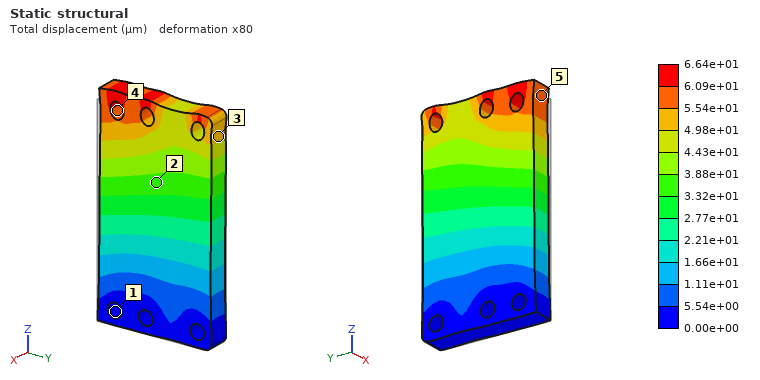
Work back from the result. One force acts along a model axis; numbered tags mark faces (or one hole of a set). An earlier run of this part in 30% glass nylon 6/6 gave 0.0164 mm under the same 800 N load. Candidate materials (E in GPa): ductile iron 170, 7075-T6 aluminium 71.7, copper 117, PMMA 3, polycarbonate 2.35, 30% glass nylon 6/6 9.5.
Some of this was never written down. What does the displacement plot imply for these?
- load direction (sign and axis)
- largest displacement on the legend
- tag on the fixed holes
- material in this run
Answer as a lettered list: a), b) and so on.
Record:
a) +Z
b) 6.64e+01 µm
c) 1
d) polycarbonate
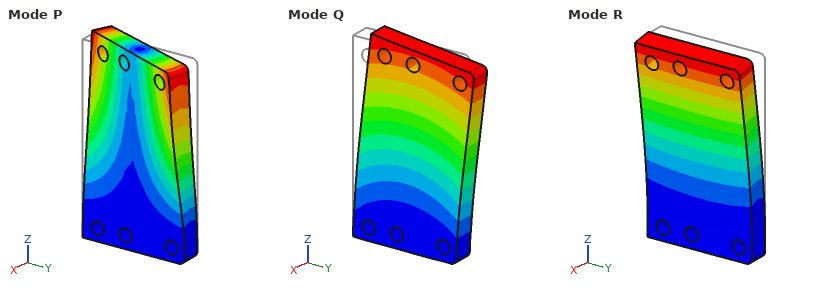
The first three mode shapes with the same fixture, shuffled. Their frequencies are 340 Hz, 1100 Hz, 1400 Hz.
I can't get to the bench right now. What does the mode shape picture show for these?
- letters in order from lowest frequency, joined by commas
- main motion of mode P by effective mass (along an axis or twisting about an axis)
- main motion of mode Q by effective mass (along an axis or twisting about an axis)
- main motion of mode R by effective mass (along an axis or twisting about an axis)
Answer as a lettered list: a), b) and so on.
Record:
a) R, P, Q
b) twisting about Z
c) along Y
d) along X
